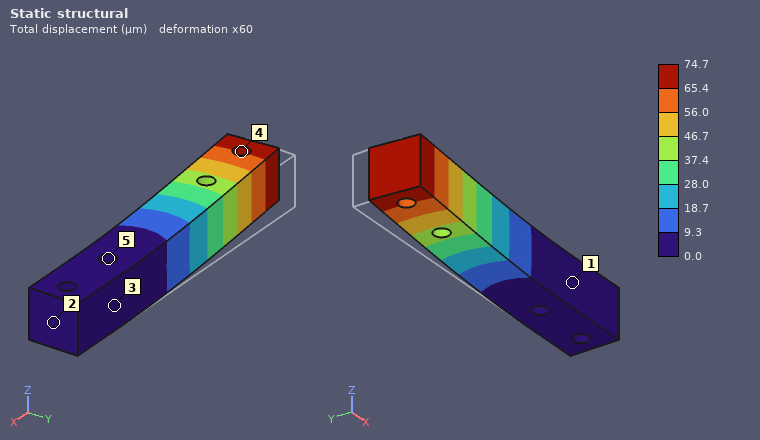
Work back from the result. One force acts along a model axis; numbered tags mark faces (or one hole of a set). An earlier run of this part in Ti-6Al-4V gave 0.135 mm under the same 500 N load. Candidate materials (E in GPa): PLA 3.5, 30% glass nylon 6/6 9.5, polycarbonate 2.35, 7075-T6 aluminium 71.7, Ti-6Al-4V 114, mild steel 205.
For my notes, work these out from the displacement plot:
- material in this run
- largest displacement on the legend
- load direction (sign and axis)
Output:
mild steel
74.7 µm
-Y
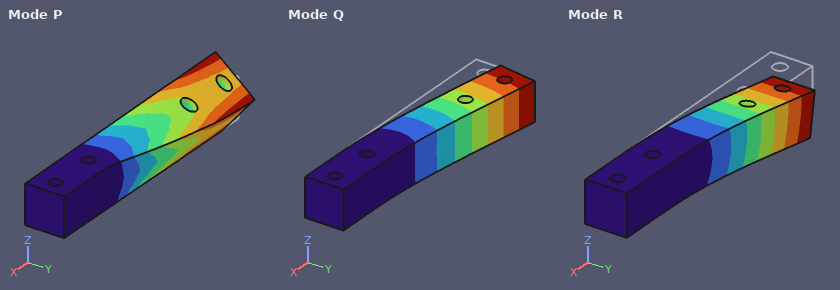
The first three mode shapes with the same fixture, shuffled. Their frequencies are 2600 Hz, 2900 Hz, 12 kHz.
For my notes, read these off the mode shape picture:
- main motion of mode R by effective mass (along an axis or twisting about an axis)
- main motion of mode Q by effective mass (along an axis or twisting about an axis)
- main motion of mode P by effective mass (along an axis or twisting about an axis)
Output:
along Z
along Y
twisting about X
